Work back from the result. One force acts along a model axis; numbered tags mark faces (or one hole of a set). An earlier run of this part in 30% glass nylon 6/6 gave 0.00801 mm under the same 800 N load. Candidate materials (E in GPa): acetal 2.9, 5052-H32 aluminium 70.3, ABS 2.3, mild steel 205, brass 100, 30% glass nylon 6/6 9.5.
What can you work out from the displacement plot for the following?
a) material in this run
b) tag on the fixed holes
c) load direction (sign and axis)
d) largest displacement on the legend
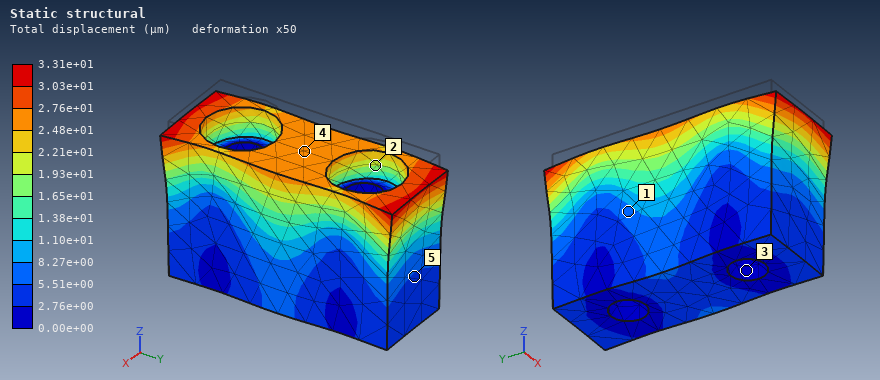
ABS
3
-Z
3.31e+01 µm
